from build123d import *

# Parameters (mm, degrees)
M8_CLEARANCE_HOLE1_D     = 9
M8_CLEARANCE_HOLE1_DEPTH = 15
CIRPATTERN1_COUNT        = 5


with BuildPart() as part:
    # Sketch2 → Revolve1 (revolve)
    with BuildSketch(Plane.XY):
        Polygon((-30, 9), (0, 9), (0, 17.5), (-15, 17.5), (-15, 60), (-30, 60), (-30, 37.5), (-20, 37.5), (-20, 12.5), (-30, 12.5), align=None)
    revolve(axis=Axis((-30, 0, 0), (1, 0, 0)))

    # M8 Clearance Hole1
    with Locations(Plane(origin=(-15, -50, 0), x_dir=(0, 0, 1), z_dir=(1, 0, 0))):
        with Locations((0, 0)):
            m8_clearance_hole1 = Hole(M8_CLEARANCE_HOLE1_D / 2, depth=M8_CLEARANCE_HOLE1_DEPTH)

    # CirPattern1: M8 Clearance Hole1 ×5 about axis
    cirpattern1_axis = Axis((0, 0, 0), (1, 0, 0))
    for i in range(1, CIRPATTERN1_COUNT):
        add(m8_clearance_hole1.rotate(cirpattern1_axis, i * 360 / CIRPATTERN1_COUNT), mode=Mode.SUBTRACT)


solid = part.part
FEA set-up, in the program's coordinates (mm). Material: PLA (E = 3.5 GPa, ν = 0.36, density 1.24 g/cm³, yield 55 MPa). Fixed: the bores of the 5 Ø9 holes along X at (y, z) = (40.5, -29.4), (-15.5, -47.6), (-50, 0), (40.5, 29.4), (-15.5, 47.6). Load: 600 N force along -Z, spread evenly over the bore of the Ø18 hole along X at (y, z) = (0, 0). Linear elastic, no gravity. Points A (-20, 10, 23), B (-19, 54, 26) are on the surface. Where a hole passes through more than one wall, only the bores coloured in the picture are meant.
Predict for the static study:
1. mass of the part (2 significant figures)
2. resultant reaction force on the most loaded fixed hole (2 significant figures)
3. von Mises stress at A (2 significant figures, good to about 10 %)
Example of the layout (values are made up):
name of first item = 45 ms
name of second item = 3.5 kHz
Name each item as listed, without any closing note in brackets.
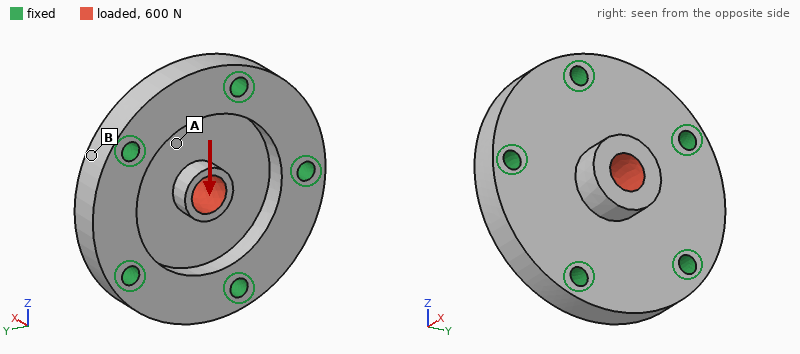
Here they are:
mass of the part = 160 g
resultant reaction force on the most loaded fixed hole = 160 N
von Mises stress at A = 0.80 MPa
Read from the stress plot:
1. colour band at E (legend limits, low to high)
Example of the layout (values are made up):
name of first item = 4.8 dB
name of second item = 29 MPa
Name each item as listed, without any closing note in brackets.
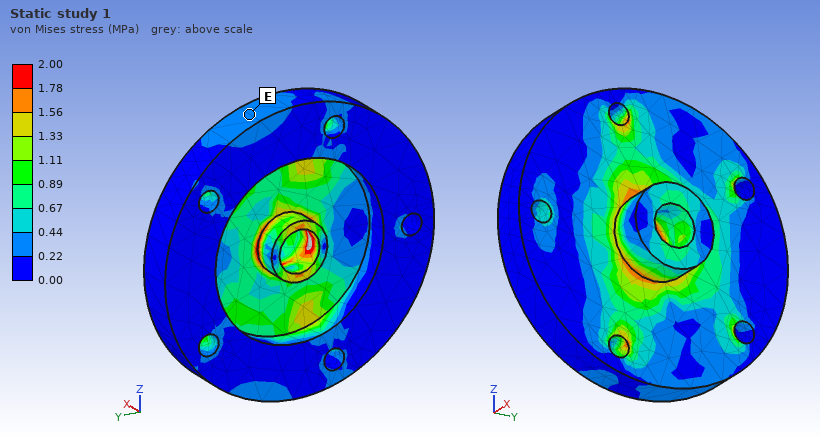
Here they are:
colour band at E = 0.22 to 0.44 MPa
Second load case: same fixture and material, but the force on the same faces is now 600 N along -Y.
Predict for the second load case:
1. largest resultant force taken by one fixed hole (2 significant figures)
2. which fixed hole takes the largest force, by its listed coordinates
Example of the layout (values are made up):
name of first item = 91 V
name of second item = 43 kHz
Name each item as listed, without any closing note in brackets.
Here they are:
largest resultant force taken by one fixed hole = 170 N
which fixed hole takes the largest force, by its listed coordinates = (-50, 0)
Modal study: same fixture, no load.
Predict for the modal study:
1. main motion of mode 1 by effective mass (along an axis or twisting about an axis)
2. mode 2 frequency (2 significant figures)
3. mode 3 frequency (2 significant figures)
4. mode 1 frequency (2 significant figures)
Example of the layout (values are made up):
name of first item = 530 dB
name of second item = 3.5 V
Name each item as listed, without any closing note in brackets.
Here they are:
main motion of mode 1 by effective mass = along X
mode 2 frequency = 3200 Hz
mode 3 frequency = 3200 Hz
mode 1 frequency = 2100 Hz
